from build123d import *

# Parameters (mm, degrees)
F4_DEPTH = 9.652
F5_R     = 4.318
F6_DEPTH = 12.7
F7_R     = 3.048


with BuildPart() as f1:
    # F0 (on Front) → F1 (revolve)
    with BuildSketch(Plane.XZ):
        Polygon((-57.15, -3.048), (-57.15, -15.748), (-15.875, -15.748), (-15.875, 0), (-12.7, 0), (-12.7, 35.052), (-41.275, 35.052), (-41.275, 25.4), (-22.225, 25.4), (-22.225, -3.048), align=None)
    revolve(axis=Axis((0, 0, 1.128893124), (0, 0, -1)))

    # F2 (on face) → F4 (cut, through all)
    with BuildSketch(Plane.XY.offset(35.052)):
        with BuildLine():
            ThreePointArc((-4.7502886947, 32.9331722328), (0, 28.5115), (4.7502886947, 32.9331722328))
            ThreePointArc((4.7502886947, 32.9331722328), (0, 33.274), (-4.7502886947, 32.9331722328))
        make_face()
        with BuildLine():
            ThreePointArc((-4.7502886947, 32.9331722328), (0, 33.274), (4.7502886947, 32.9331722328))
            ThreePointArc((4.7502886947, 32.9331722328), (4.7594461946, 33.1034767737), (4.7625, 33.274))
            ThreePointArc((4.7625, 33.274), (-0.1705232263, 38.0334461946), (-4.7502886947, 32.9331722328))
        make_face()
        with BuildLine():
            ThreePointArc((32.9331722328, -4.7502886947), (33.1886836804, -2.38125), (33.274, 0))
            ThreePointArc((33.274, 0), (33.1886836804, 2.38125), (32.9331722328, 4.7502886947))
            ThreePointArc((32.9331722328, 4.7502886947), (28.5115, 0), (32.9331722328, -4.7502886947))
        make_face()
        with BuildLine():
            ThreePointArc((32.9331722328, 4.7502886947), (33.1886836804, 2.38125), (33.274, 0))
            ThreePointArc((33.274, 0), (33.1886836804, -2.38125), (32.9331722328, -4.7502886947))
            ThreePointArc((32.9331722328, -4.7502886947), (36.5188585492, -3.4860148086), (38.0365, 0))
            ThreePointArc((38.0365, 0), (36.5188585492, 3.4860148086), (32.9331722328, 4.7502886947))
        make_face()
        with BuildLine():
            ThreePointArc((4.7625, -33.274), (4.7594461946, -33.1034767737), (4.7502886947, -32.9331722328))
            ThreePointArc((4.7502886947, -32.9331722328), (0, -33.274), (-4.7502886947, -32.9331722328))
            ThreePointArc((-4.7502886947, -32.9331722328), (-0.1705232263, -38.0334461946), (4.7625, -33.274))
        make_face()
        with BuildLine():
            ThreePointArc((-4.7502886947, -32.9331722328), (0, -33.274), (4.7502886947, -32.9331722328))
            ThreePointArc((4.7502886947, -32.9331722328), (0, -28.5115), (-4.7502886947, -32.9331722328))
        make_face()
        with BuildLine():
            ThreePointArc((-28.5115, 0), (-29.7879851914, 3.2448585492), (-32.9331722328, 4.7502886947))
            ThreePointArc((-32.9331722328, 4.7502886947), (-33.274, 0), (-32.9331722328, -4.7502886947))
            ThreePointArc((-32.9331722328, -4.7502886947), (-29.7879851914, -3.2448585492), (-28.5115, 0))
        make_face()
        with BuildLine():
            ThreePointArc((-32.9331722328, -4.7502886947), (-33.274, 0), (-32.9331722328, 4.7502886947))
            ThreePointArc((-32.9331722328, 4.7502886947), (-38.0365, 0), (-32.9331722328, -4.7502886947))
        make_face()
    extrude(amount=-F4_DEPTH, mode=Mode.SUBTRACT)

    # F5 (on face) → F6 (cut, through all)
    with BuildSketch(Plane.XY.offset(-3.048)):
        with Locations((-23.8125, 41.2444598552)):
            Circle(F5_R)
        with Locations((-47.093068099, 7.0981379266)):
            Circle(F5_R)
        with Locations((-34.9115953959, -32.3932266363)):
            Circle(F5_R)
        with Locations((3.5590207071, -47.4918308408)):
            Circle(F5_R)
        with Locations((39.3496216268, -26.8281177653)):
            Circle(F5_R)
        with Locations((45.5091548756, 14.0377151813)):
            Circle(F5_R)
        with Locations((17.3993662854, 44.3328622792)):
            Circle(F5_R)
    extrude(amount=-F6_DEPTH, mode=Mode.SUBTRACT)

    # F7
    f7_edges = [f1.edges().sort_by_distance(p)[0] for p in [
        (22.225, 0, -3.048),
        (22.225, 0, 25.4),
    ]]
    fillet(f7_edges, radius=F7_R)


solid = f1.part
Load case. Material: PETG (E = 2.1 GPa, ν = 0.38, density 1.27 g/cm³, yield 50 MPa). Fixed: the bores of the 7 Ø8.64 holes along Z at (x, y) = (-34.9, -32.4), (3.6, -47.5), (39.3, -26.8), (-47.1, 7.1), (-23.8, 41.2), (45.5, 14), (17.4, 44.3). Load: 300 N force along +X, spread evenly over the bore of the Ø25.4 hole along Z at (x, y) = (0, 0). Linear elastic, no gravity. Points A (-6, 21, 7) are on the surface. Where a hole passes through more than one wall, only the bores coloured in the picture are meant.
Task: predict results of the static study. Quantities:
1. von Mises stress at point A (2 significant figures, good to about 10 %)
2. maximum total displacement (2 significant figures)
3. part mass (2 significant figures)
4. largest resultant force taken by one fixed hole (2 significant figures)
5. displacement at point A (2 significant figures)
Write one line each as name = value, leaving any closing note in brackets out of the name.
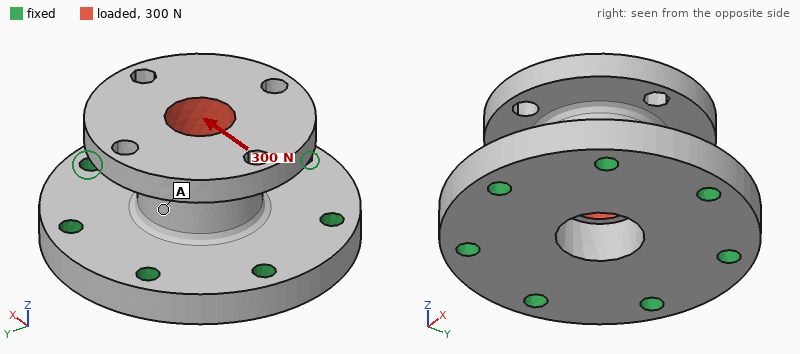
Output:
von Mises stress at point A = 0.40 MPa
maximum total displacement = 58 µm
part mass = 240 g
largest resultant force taken by one fixed hole = 94 N
displacement at point A = 17 µm
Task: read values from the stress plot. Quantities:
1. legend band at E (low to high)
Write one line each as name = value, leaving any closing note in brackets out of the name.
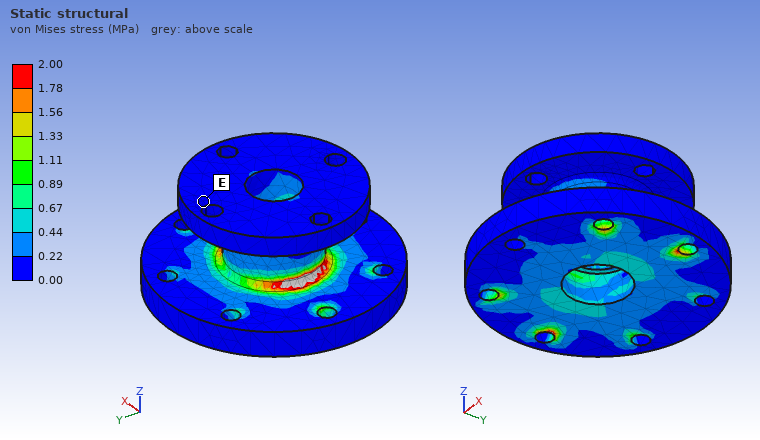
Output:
legend band at E = 0.00 to 0.22 MPa
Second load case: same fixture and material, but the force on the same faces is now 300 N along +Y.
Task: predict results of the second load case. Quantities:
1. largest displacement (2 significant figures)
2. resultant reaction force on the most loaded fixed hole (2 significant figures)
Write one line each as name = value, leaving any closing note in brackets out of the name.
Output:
largest displacement = 58 µm
resultant reaction force on the most loaded fixed hole = 95 N
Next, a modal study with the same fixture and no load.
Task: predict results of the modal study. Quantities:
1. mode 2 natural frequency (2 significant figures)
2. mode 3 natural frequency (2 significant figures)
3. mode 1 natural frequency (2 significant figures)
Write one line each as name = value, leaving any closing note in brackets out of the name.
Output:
mode 2 natural frequency = 1100 Hz
mode 3 natural frequency = 1700 Hz
mode 1 natural frequency = 1100 Hz
